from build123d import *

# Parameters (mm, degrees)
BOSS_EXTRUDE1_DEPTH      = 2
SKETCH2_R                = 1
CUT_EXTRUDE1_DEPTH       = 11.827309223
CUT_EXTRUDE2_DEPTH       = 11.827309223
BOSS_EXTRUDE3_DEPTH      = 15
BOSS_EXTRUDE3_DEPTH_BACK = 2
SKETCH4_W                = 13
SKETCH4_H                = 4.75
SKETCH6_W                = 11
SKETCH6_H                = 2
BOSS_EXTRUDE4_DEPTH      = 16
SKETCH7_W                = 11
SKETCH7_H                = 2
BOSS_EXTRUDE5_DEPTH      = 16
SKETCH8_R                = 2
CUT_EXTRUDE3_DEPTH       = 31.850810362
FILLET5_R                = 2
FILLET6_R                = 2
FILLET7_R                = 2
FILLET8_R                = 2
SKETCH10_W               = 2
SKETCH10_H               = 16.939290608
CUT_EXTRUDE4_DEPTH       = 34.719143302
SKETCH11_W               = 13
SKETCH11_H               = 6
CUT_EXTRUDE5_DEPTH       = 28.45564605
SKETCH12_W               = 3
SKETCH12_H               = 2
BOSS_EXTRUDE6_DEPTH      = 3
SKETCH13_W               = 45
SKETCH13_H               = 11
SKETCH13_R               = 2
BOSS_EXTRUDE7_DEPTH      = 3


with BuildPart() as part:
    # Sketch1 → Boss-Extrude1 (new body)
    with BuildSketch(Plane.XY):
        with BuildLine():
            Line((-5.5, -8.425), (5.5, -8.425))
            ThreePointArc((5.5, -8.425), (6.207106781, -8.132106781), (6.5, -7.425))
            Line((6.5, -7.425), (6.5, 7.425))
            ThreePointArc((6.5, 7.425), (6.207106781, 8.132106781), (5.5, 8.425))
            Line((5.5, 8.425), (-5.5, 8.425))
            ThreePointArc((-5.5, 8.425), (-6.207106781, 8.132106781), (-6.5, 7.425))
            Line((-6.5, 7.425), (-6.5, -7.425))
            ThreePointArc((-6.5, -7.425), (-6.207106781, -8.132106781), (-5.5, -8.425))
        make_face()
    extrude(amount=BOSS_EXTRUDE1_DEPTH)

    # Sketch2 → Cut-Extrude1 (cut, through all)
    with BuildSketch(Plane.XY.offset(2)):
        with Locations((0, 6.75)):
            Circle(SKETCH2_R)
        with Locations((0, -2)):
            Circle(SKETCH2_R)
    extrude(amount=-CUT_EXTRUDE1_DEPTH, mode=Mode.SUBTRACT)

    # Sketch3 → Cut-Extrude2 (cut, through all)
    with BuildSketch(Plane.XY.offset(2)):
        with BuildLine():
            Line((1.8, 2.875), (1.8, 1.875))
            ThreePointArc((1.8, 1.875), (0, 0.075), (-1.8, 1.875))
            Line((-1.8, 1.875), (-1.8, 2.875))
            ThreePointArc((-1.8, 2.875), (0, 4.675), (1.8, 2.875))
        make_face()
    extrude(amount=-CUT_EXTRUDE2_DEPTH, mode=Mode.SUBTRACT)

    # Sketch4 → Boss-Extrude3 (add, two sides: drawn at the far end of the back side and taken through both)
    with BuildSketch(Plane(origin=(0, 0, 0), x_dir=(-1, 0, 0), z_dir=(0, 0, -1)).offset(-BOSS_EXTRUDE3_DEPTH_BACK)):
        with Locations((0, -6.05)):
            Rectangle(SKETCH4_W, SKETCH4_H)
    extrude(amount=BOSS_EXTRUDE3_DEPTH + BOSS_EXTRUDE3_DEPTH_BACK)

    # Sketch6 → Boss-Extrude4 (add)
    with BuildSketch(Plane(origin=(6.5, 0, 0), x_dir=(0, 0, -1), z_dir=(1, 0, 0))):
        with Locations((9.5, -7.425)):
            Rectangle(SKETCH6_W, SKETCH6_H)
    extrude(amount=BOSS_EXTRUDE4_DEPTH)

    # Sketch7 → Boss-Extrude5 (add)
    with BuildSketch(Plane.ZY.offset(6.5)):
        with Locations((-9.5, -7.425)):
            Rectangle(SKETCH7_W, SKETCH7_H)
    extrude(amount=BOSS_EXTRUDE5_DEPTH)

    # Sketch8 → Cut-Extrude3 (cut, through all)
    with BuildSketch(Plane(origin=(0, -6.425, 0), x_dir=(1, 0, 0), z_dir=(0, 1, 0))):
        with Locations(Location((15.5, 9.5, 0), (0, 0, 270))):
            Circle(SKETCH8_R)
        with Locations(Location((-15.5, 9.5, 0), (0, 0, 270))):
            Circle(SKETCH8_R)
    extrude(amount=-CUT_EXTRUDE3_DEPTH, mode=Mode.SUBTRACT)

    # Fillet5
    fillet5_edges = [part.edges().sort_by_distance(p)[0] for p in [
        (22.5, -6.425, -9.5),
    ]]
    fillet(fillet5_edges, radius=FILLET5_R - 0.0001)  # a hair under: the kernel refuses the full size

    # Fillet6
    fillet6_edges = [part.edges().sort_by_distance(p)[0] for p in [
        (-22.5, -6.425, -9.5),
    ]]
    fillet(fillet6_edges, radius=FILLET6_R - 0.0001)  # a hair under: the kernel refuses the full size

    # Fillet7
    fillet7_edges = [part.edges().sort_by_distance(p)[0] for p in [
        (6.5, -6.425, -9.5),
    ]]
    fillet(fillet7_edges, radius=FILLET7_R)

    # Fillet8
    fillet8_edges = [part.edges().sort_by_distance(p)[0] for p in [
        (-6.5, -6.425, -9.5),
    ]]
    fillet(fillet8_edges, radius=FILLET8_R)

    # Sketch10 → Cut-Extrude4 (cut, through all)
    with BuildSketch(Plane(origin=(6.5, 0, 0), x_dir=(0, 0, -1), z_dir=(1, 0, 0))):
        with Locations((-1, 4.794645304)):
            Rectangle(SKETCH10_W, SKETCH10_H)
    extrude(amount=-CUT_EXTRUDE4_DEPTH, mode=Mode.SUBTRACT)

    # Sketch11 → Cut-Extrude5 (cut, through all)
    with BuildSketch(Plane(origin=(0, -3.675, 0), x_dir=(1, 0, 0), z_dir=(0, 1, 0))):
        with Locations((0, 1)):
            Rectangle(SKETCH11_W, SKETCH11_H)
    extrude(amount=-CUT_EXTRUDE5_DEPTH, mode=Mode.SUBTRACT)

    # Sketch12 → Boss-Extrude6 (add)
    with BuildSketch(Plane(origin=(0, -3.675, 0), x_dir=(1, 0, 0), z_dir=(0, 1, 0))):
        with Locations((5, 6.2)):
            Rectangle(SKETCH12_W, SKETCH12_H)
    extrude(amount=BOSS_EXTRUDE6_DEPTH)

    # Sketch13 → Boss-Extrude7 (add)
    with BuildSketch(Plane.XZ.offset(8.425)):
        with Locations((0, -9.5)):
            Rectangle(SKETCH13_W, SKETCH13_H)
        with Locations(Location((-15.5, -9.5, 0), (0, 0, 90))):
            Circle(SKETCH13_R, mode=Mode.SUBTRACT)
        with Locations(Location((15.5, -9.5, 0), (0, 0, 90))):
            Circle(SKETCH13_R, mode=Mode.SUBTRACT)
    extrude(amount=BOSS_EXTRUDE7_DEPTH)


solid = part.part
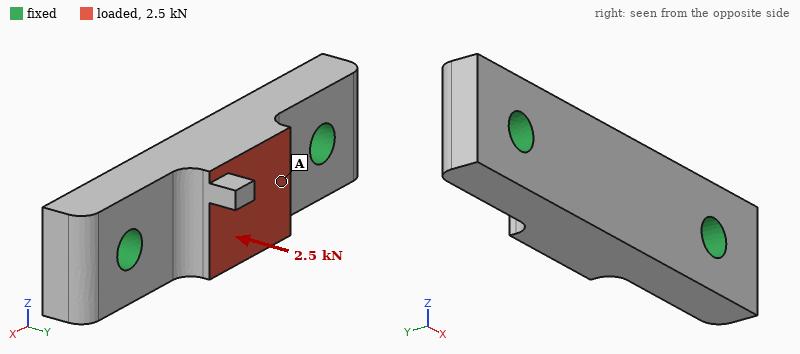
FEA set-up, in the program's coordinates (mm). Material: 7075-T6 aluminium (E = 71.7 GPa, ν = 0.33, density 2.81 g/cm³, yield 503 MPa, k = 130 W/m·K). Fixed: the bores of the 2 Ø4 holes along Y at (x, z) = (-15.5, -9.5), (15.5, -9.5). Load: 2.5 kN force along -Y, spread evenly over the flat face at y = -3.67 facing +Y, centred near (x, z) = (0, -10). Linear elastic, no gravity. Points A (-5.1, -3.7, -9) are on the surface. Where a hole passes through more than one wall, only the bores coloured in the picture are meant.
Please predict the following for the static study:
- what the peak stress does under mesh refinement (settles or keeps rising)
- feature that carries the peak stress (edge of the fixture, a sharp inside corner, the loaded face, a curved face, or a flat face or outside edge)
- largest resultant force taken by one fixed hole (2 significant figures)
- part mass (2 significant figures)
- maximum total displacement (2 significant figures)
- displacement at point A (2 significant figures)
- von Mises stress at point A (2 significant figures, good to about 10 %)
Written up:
keeps rising
edge of the fixture
1.4 kN
7.8 g
28 µm
23 µm
32 MPa
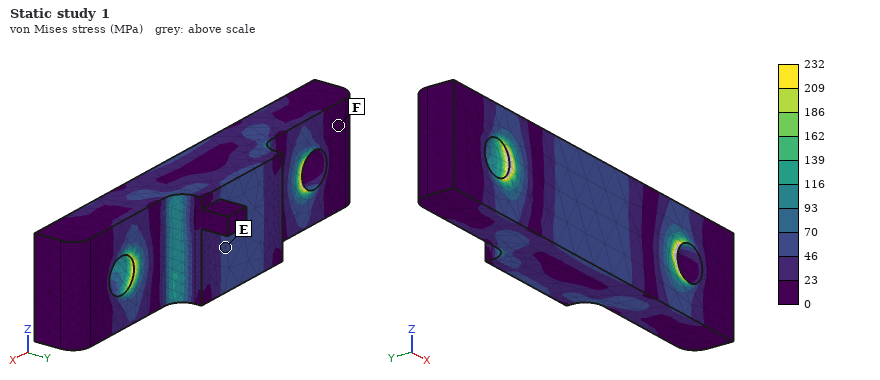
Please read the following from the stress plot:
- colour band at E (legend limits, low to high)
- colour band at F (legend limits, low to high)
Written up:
46 to 70 MPa
0 to 23 MPa
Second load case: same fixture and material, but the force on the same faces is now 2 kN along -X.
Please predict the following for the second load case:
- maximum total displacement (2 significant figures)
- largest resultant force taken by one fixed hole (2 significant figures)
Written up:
8.9 µm
1.1 kN
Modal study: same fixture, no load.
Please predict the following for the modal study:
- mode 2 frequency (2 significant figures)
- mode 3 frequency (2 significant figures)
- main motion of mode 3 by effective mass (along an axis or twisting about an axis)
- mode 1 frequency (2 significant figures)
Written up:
26 kHz
35 kHz
along Z
26 kHz
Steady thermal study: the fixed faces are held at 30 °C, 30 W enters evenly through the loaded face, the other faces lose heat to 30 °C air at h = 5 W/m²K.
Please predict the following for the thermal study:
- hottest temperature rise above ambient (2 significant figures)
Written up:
28 K
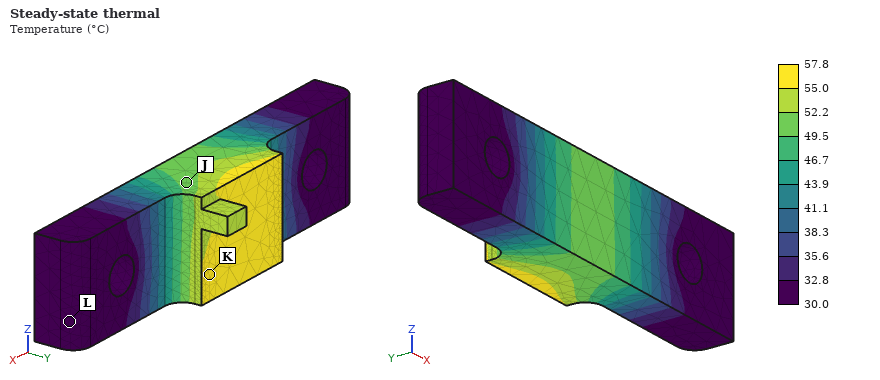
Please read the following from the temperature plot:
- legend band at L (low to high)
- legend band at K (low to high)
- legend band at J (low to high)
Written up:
30.0 to 32.8 °C
55.0 to 57.8 °C
49.5 to 52.2 °C
